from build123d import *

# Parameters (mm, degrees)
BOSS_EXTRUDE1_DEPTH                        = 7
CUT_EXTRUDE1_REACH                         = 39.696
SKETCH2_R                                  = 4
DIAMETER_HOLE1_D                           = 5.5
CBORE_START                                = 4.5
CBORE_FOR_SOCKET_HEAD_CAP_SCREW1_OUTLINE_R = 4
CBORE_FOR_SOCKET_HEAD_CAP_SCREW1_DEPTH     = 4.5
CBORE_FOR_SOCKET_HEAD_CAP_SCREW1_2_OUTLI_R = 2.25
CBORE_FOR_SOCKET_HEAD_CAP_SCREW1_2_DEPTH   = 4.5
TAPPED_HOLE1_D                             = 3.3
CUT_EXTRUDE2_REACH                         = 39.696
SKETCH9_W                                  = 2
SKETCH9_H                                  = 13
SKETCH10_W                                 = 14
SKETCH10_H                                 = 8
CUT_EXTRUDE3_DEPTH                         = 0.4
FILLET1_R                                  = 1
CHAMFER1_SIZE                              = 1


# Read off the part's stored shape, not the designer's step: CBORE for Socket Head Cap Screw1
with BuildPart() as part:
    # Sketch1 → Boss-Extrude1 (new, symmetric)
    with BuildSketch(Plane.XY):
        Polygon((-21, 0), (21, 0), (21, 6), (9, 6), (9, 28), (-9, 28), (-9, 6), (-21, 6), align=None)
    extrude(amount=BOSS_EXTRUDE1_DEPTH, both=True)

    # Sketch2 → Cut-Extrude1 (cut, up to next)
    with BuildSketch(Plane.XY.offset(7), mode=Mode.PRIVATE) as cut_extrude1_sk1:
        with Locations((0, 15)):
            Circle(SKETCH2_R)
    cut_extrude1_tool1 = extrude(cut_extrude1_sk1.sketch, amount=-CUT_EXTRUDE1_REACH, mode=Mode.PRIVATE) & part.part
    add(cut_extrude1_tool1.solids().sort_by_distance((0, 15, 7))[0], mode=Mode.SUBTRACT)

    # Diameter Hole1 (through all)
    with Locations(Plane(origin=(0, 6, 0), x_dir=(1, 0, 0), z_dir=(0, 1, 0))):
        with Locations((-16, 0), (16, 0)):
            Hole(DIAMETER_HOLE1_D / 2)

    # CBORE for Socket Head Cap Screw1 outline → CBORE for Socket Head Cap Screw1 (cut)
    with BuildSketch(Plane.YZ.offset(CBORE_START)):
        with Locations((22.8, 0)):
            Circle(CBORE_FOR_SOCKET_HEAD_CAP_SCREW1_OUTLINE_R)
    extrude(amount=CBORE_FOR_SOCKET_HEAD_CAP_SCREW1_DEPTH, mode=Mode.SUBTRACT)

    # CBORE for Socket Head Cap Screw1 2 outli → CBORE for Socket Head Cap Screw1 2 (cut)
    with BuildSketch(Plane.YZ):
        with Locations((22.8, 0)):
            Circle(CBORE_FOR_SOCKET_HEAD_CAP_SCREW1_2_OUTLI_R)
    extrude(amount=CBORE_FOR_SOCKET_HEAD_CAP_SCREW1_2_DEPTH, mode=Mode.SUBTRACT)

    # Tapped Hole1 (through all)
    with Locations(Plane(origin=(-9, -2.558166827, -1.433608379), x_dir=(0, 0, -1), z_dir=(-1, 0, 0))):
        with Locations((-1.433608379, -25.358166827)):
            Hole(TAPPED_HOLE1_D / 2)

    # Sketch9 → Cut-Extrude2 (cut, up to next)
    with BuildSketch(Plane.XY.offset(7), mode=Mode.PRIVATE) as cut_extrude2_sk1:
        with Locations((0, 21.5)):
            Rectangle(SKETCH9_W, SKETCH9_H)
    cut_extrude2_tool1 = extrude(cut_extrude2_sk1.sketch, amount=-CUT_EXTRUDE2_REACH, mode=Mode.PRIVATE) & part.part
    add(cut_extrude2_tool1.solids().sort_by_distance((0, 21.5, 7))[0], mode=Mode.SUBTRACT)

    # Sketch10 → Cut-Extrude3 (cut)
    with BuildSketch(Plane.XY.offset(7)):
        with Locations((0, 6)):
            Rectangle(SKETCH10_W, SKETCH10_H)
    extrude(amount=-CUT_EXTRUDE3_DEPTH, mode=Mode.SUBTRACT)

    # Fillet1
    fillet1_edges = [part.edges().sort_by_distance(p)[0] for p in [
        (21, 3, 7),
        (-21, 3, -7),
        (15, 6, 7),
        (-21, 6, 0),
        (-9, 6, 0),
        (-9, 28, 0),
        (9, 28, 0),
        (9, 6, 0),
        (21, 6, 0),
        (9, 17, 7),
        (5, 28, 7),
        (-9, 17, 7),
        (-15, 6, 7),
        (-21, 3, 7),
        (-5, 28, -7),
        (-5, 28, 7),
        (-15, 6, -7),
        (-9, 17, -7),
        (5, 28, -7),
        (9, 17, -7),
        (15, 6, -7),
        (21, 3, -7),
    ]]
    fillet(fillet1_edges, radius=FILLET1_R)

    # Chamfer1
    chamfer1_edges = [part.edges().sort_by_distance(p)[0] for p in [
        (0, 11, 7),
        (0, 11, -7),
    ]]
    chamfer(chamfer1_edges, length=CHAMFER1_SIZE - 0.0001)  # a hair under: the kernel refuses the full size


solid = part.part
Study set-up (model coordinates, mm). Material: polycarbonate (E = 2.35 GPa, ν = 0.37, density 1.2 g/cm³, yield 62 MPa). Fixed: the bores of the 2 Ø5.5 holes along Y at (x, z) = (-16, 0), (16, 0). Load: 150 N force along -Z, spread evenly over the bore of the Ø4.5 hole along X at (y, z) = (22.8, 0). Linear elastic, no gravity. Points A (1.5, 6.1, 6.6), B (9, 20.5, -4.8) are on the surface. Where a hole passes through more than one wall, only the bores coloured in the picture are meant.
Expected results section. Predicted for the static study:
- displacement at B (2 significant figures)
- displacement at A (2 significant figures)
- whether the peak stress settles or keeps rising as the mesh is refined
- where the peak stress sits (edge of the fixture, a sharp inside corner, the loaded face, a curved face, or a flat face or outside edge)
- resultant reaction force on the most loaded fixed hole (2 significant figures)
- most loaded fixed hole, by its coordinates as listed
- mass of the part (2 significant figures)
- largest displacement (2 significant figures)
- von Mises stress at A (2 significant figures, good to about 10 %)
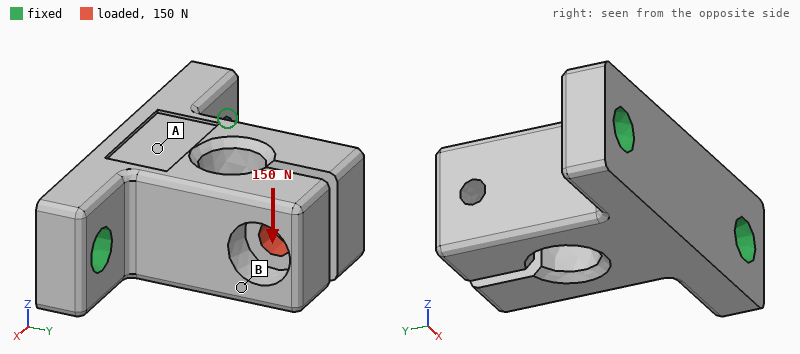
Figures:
0.36 mm
0.11 mm
keeps rising
edge of the fixture
88 N
(16, 0)
8.8 g
0.61 mm
5.1 MPa
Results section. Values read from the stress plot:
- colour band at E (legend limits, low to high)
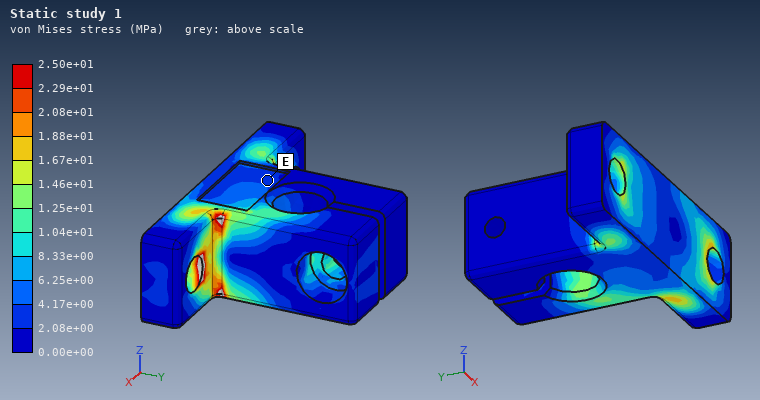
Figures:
2.08e+00 to 4.17e+00 MPa
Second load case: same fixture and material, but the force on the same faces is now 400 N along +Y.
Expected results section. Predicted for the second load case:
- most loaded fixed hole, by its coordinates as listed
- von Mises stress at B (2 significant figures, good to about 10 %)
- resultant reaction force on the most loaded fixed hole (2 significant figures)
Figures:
(16, 0)
7.2 MPa
270 N
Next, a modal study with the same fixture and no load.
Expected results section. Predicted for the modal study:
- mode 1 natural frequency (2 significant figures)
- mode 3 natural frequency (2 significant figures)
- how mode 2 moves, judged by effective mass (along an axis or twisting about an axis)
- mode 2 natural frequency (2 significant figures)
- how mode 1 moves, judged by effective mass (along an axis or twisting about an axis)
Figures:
1900 Hz
2800 Hz
along X
2600 Hz
along Z
